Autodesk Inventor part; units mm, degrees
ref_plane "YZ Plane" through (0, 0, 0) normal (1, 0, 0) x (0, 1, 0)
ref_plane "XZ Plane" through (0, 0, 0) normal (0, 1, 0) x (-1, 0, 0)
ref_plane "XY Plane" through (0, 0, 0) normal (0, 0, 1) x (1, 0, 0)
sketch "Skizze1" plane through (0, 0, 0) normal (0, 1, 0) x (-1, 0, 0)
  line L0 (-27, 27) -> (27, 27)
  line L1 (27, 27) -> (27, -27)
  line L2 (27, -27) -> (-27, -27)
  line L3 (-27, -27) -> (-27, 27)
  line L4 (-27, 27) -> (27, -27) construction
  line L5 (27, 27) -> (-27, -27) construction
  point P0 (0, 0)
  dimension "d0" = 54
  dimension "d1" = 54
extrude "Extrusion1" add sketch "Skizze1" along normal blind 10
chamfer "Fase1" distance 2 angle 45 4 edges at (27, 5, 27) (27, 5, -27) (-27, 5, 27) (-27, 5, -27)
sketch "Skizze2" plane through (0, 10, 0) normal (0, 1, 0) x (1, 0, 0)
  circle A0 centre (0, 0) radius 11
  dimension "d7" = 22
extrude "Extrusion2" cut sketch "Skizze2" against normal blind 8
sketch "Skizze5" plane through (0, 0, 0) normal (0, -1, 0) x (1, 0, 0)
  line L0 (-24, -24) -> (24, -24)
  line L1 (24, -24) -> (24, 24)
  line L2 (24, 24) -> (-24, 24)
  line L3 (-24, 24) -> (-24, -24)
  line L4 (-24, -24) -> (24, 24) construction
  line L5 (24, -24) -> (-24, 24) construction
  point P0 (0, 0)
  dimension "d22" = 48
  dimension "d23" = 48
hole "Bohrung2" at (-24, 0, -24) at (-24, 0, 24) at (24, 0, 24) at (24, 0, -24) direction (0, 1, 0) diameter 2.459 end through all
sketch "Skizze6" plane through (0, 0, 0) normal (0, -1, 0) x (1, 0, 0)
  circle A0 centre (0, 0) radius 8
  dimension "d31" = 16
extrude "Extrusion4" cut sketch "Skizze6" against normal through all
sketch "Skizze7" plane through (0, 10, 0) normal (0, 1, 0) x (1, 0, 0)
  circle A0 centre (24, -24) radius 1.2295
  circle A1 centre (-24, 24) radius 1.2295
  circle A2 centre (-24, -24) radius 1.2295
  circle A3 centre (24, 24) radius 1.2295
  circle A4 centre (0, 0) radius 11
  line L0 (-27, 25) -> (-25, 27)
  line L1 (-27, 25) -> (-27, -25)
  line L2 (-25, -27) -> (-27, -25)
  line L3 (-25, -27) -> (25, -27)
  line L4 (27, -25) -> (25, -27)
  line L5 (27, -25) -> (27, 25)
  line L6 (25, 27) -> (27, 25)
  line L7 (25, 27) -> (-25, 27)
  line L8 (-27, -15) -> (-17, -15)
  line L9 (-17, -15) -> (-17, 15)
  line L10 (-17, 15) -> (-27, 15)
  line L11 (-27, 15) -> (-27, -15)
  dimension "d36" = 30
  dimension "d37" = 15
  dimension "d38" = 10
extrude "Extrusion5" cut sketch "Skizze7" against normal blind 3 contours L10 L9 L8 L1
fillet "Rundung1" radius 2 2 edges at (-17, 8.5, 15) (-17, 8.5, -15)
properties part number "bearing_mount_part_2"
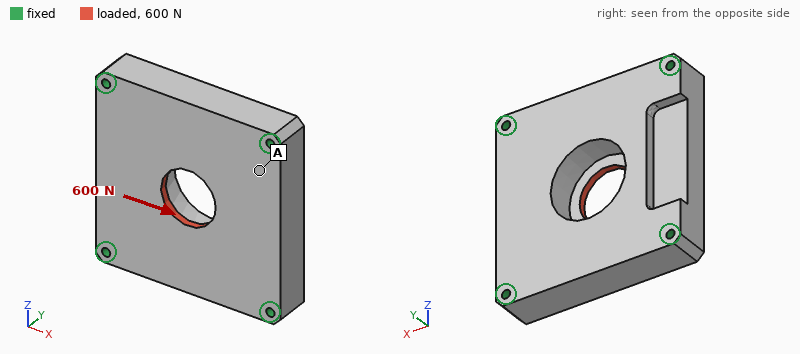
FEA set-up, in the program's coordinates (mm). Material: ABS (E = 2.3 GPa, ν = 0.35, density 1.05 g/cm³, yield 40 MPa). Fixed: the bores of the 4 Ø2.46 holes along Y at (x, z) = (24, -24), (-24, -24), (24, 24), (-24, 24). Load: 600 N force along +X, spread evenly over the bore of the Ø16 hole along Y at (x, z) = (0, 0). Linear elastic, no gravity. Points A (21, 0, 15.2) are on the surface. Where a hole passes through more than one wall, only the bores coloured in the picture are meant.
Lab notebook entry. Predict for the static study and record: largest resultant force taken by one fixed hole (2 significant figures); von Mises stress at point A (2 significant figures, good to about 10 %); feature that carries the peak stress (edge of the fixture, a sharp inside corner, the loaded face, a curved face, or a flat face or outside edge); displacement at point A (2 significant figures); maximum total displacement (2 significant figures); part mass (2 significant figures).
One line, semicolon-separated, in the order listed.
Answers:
170 N; 1.7 MPa; a sharp inside corner; 14 µm; 49 µm; 26 g
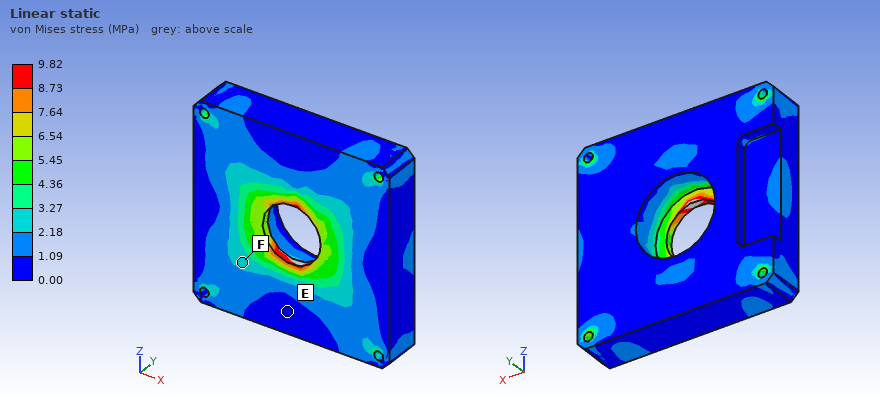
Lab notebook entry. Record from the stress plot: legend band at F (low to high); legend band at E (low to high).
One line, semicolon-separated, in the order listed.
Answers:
2.18 to 3.27 MPa; 0.00 to 1.09 MPa
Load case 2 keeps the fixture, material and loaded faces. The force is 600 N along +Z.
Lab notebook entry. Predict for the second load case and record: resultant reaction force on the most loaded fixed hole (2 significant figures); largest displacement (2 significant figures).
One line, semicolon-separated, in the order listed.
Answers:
180 N; 50 µm
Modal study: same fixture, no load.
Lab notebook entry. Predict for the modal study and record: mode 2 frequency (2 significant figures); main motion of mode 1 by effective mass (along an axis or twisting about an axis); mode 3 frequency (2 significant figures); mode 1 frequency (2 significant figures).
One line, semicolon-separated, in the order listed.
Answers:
4900 Hz; along Y; 5000 Hz; 3300 Hz
